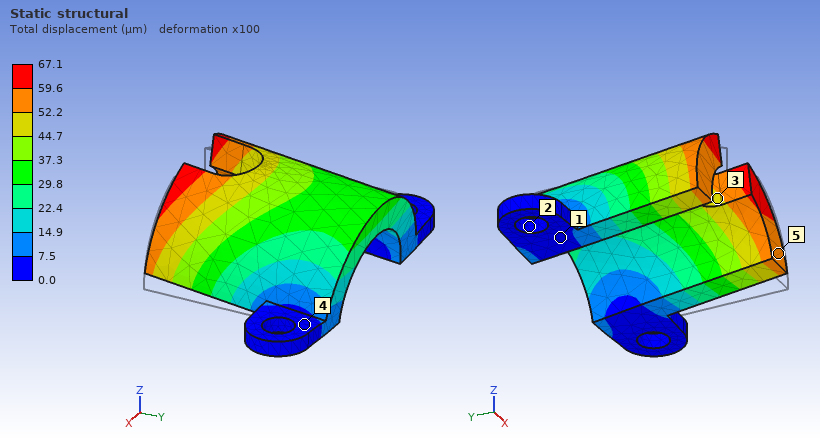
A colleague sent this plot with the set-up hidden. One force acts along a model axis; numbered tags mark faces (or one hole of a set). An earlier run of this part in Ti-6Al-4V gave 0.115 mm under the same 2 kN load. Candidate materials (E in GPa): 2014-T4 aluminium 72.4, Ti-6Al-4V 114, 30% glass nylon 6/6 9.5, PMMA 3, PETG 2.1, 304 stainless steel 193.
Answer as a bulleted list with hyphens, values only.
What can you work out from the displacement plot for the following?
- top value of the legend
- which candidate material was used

- 67.1 µm
- 304 stainless steel
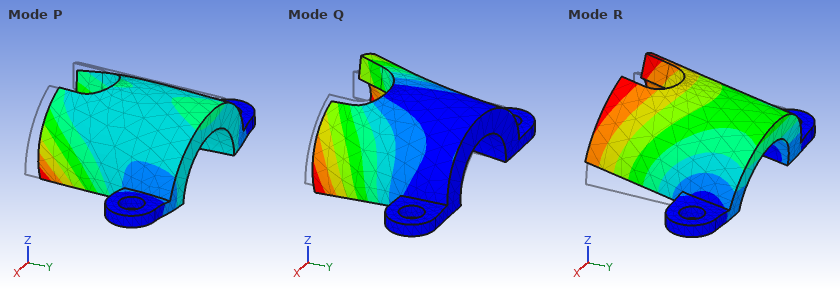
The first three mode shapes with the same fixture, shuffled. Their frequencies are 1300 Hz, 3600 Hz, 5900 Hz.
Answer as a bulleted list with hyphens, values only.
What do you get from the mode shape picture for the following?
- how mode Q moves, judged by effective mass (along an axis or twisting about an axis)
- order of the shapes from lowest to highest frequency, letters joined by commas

- along X
- R, Q, P
